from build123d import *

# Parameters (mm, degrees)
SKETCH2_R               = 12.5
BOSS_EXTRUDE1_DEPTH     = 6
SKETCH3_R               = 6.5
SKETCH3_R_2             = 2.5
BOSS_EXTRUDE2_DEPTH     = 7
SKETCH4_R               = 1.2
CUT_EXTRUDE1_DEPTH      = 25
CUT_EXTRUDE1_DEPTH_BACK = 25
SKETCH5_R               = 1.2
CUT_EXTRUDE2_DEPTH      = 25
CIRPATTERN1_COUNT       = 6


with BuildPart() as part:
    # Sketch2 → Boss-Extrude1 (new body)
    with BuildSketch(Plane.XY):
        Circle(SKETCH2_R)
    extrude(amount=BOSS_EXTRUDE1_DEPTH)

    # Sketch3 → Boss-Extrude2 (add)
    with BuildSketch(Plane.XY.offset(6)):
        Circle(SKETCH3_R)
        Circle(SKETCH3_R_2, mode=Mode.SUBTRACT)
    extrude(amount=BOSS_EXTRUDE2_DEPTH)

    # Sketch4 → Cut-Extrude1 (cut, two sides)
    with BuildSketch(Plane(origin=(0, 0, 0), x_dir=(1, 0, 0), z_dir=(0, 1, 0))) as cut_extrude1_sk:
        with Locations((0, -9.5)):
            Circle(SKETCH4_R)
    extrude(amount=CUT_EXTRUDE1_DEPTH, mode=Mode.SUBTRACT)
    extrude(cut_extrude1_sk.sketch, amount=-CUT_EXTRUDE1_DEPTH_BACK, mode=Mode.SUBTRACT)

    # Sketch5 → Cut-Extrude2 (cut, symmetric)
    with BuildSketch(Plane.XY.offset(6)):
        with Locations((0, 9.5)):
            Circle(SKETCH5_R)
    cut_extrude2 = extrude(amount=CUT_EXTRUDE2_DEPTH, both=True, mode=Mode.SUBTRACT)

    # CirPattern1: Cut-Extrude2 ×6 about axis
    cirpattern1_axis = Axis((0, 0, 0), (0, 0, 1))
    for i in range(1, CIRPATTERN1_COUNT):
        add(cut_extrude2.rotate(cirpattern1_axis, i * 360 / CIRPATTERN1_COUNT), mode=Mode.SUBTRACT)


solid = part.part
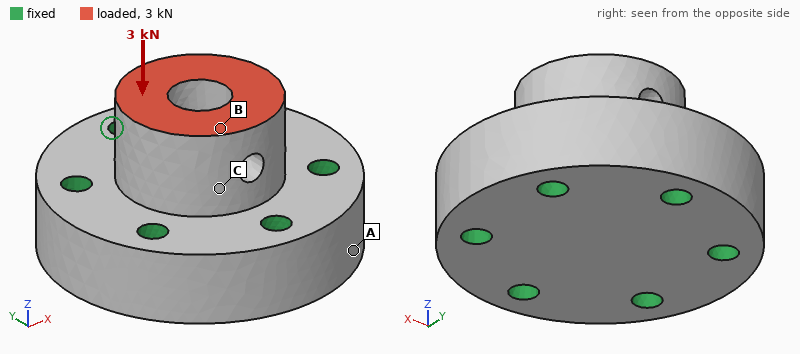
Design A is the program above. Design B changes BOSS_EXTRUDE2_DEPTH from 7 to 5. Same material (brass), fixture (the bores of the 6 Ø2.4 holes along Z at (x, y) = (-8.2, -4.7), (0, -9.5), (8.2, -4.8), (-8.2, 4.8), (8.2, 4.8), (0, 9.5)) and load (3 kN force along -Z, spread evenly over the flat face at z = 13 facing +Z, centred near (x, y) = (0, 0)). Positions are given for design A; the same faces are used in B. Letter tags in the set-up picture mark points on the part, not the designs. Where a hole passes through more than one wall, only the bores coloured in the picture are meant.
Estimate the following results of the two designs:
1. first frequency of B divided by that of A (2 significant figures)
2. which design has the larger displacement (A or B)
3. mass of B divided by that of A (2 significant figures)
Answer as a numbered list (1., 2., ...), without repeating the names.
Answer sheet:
1. 1.4
2. B
3. 0.94
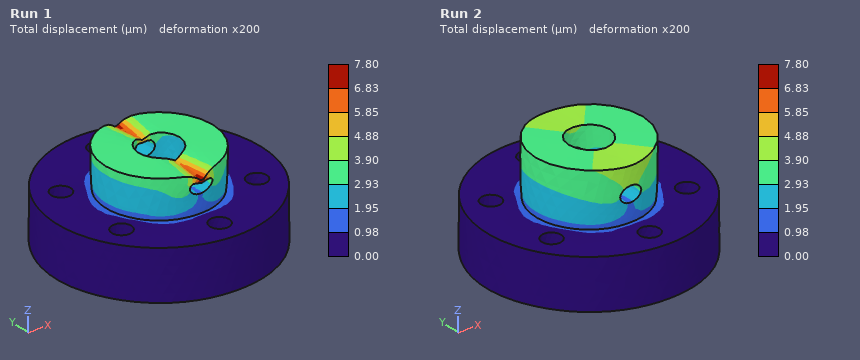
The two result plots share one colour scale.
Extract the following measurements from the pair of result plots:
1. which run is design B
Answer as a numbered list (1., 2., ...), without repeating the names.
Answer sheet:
1. Run 1
